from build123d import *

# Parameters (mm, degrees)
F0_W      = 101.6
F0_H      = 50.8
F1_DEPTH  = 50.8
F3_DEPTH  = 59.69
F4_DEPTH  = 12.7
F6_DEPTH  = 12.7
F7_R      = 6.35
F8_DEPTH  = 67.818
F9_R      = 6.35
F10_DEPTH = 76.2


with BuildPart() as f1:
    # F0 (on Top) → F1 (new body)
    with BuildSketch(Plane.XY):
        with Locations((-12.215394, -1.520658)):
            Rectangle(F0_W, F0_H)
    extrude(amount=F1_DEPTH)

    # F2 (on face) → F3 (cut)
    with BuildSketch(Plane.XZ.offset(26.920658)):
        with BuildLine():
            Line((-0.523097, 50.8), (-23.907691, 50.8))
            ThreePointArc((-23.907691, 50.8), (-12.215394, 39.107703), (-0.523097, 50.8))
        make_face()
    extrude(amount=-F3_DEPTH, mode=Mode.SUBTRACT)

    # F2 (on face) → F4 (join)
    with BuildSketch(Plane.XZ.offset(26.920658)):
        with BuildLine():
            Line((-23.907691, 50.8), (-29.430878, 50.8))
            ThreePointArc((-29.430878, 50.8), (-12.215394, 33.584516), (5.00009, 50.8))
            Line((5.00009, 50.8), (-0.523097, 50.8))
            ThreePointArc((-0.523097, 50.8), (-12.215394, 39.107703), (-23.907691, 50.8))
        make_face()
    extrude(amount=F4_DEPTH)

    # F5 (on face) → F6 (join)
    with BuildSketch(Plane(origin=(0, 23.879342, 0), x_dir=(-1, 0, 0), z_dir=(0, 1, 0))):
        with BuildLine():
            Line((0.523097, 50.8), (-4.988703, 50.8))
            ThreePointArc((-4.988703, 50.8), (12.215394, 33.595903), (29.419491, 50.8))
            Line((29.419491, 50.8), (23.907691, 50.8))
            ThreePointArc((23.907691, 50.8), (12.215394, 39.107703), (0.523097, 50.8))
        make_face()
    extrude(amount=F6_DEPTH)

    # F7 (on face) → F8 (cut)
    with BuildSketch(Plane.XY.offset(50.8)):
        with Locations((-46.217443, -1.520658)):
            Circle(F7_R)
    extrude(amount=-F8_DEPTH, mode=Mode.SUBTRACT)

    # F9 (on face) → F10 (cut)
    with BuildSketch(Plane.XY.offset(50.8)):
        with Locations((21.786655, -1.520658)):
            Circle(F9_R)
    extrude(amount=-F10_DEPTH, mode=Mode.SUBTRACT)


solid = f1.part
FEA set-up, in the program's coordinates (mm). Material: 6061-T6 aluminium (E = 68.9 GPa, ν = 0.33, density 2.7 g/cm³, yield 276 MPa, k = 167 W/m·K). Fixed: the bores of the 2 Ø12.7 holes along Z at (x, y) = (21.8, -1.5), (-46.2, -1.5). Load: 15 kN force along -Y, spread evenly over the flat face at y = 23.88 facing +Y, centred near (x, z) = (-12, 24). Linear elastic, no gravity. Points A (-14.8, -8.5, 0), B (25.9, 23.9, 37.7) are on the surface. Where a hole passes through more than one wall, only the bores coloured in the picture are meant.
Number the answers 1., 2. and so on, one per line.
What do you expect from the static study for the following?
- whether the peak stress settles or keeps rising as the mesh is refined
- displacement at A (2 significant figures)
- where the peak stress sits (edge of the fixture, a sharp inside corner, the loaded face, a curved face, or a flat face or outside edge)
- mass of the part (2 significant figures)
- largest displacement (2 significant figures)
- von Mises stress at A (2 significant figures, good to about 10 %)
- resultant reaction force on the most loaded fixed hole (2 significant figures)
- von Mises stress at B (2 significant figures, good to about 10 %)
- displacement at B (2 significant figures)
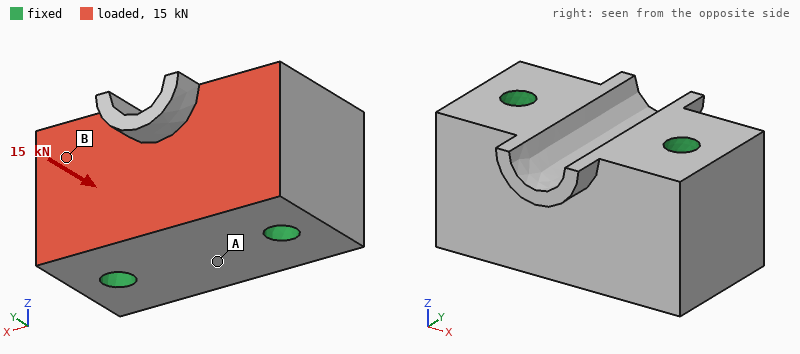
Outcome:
1. keeps rising
2. 1.8 µm
3. edge of the fixture
4. 660 g
5. 2.9 µm
6. 1.2 MPa
7. 7.5 kN
8. 3.9 MPa
9. 1.1 µm
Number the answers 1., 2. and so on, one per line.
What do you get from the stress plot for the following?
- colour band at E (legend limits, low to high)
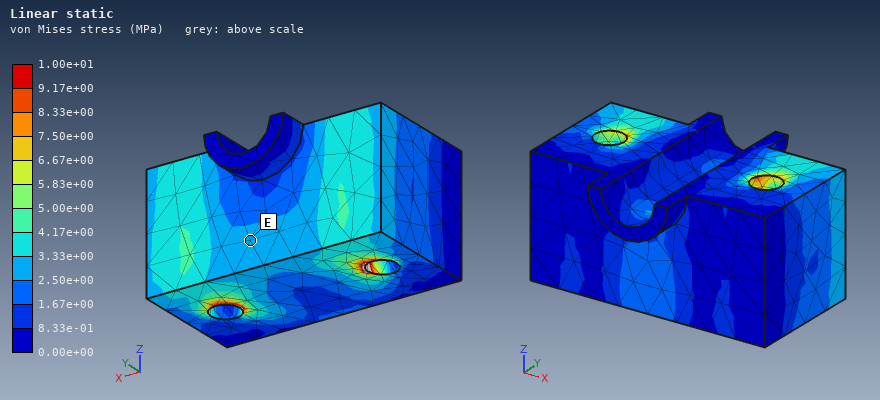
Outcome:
1. 2.50e+00 to 3.33e+00 MPa
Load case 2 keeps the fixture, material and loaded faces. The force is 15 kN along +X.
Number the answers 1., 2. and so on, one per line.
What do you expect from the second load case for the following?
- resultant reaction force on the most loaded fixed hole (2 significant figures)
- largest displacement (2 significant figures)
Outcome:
1. 8.6 kN
2. 6.4 µm
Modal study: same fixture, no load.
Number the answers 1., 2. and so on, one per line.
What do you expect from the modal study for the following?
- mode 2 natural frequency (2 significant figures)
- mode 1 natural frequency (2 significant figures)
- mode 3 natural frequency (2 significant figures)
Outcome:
1. 18 kHz
2. 18 kHz
3. 18 kHz
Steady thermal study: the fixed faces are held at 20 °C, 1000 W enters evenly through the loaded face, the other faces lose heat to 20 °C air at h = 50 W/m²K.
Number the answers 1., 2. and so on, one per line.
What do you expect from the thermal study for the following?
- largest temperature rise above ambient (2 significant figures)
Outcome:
1. 38 K
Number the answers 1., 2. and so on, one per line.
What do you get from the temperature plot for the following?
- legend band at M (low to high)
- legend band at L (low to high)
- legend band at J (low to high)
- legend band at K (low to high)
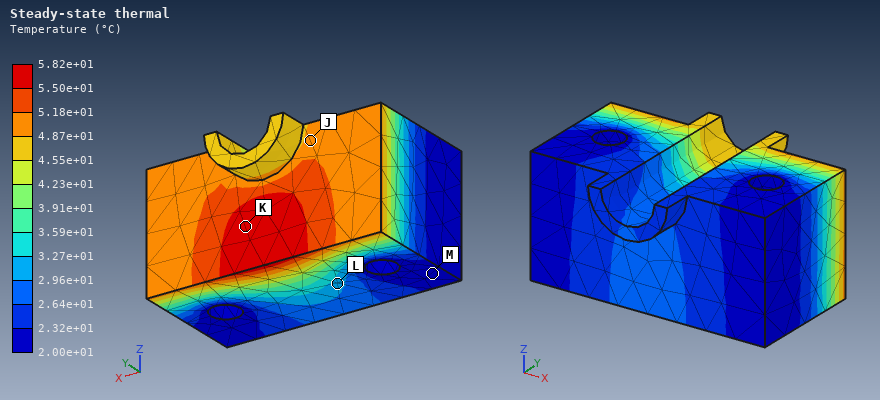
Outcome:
1. 2.00e+01 to 2.32e+01 °C
2. 2.96e+01 to 3.27e+01 °C
3. 4.87e+01 to 5.18e+01 °C
4. 5.50e+01 to 5.82e+01 °C
